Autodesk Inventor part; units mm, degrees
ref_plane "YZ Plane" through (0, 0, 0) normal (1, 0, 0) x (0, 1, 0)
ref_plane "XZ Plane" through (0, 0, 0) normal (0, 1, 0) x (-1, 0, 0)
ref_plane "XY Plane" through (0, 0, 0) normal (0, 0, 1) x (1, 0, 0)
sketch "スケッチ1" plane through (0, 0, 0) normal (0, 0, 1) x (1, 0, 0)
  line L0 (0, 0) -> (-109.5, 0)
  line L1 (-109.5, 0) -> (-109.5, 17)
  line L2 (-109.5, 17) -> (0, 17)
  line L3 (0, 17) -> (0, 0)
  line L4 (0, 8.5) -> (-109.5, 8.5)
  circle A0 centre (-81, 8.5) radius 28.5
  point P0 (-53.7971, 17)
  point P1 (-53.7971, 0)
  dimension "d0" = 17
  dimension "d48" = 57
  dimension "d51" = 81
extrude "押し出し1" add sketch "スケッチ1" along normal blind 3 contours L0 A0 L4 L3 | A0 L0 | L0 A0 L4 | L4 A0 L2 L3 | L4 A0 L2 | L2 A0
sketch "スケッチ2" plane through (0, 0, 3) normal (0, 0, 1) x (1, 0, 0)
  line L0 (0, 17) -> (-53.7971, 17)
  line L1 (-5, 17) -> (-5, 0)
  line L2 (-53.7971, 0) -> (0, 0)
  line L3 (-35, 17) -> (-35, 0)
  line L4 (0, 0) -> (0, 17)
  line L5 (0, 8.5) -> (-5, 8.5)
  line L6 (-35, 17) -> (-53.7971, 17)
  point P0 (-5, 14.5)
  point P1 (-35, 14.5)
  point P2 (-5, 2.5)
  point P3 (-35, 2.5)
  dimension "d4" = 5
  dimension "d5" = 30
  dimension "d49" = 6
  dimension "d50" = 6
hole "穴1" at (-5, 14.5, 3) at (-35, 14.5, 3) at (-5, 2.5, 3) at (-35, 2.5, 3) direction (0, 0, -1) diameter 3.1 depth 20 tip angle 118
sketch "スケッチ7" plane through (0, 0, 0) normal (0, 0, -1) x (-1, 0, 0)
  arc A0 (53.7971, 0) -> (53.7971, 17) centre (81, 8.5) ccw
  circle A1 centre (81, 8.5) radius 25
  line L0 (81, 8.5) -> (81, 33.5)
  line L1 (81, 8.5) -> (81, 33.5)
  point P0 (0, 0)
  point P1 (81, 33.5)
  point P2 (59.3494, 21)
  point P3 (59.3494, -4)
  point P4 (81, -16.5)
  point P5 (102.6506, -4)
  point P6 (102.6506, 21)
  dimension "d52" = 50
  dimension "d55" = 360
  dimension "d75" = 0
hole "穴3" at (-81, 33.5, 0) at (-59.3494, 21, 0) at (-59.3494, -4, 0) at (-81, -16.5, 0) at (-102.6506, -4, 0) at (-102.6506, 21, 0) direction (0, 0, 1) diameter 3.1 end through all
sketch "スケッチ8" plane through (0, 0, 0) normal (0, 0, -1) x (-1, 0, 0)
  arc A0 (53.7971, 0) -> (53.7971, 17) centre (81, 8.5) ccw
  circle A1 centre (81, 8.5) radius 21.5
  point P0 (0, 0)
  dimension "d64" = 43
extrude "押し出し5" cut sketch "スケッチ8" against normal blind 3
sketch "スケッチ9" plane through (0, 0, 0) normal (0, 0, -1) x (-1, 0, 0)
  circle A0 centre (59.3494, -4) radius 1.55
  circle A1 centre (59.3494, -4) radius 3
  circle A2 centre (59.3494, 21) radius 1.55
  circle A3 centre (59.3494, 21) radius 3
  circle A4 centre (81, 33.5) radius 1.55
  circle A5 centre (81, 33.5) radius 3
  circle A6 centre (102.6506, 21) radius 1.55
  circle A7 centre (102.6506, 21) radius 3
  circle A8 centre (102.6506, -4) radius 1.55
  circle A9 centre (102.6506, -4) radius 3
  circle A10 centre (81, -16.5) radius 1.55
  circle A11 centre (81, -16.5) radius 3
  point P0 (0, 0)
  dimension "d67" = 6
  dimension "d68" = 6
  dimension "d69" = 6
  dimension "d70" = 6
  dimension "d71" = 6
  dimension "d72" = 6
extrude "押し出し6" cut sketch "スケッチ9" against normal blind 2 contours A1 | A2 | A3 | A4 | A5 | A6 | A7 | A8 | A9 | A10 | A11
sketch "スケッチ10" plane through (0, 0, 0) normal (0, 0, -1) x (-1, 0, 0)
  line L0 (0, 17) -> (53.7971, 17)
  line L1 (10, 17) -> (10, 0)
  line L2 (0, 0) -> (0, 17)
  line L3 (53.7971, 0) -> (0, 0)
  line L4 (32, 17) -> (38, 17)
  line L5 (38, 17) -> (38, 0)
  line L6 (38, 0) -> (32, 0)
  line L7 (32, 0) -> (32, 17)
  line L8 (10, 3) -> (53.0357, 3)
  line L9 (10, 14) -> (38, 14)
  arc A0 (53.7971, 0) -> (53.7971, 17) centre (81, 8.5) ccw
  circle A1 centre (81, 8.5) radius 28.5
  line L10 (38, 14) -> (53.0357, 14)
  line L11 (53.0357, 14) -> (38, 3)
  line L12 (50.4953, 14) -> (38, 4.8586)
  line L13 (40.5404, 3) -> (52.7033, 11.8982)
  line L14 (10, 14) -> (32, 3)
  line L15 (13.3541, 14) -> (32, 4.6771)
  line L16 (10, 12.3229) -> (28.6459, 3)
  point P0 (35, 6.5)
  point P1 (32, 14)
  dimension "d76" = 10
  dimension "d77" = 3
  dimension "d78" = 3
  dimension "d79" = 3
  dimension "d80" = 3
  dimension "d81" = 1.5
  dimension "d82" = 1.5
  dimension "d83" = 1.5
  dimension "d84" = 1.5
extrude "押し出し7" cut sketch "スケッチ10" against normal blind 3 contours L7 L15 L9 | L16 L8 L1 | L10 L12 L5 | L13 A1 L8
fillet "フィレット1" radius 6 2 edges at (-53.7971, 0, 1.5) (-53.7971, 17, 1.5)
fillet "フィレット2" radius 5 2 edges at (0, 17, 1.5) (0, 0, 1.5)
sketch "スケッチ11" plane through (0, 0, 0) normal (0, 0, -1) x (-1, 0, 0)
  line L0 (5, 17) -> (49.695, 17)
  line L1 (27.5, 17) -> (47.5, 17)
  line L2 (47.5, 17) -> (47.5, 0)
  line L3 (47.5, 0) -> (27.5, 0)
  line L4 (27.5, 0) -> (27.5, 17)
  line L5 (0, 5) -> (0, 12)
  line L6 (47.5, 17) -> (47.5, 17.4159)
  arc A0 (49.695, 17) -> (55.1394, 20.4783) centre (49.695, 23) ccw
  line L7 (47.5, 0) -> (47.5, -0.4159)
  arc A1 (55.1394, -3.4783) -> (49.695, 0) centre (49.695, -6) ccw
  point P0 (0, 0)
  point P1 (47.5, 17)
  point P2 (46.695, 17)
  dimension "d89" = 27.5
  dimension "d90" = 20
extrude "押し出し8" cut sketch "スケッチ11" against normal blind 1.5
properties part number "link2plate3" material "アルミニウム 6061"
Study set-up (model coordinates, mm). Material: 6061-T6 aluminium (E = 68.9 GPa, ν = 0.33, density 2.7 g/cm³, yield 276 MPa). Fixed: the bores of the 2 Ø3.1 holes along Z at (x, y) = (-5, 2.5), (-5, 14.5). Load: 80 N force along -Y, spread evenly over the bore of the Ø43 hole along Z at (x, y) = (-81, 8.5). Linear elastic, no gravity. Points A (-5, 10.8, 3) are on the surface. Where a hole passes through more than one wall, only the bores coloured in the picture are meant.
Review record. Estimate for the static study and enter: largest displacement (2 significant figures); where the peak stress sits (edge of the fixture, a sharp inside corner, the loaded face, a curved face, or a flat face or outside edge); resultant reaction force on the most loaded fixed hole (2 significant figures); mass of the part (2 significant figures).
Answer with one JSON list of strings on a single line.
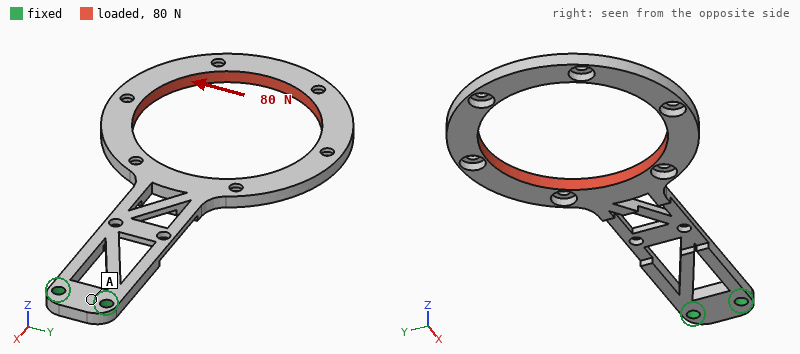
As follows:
["0.59 mm", "a curved face", "450 N", "12 g"]
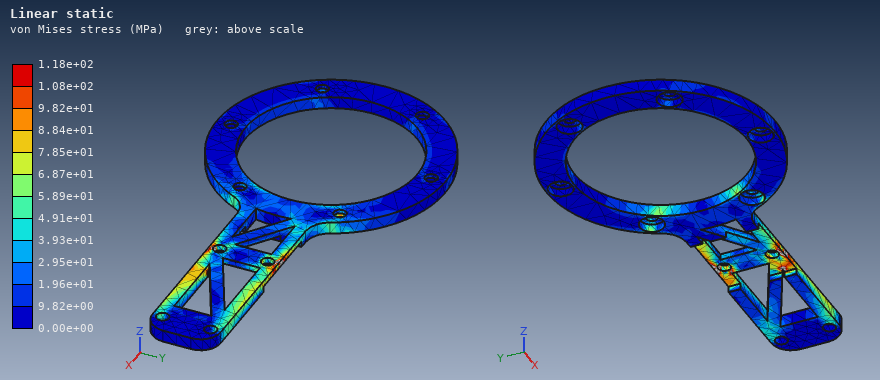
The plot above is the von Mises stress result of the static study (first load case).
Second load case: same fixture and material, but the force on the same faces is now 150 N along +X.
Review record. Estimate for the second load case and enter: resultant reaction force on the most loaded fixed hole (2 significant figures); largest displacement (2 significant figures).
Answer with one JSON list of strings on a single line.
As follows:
["77 N", "1.2 mm"]
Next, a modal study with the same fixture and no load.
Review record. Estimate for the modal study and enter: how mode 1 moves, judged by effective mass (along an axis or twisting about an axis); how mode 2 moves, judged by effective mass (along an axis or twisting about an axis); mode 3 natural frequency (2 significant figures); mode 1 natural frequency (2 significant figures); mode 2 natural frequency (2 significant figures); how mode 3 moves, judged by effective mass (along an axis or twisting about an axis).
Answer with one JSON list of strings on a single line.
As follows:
["along Z", "twisting about X", "750 Hz", "89 Hz", "320 Hz", "along Y"]
